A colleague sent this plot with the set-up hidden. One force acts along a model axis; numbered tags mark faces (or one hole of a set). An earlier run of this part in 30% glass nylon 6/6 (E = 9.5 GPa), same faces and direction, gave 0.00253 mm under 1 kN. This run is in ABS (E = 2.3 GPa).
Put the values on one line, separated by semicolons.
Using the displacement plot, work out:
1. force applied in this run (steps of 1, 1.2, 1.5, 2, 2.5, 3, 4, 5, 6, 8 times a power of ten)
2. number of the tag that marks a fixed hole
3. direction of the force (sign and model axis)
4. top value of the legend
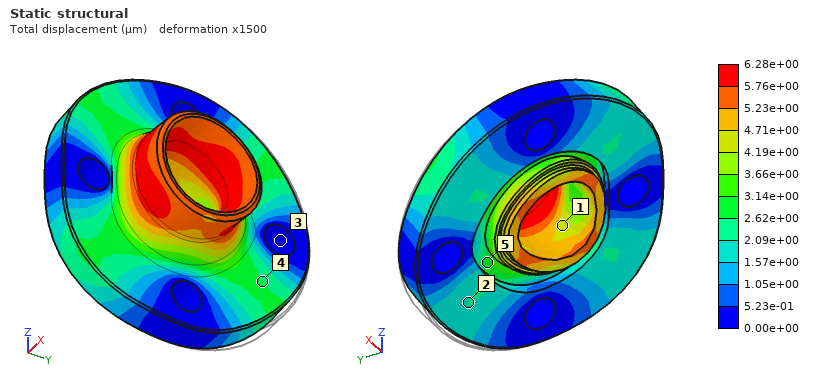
600 N; 3; -Y; 6.28e+00 µm
